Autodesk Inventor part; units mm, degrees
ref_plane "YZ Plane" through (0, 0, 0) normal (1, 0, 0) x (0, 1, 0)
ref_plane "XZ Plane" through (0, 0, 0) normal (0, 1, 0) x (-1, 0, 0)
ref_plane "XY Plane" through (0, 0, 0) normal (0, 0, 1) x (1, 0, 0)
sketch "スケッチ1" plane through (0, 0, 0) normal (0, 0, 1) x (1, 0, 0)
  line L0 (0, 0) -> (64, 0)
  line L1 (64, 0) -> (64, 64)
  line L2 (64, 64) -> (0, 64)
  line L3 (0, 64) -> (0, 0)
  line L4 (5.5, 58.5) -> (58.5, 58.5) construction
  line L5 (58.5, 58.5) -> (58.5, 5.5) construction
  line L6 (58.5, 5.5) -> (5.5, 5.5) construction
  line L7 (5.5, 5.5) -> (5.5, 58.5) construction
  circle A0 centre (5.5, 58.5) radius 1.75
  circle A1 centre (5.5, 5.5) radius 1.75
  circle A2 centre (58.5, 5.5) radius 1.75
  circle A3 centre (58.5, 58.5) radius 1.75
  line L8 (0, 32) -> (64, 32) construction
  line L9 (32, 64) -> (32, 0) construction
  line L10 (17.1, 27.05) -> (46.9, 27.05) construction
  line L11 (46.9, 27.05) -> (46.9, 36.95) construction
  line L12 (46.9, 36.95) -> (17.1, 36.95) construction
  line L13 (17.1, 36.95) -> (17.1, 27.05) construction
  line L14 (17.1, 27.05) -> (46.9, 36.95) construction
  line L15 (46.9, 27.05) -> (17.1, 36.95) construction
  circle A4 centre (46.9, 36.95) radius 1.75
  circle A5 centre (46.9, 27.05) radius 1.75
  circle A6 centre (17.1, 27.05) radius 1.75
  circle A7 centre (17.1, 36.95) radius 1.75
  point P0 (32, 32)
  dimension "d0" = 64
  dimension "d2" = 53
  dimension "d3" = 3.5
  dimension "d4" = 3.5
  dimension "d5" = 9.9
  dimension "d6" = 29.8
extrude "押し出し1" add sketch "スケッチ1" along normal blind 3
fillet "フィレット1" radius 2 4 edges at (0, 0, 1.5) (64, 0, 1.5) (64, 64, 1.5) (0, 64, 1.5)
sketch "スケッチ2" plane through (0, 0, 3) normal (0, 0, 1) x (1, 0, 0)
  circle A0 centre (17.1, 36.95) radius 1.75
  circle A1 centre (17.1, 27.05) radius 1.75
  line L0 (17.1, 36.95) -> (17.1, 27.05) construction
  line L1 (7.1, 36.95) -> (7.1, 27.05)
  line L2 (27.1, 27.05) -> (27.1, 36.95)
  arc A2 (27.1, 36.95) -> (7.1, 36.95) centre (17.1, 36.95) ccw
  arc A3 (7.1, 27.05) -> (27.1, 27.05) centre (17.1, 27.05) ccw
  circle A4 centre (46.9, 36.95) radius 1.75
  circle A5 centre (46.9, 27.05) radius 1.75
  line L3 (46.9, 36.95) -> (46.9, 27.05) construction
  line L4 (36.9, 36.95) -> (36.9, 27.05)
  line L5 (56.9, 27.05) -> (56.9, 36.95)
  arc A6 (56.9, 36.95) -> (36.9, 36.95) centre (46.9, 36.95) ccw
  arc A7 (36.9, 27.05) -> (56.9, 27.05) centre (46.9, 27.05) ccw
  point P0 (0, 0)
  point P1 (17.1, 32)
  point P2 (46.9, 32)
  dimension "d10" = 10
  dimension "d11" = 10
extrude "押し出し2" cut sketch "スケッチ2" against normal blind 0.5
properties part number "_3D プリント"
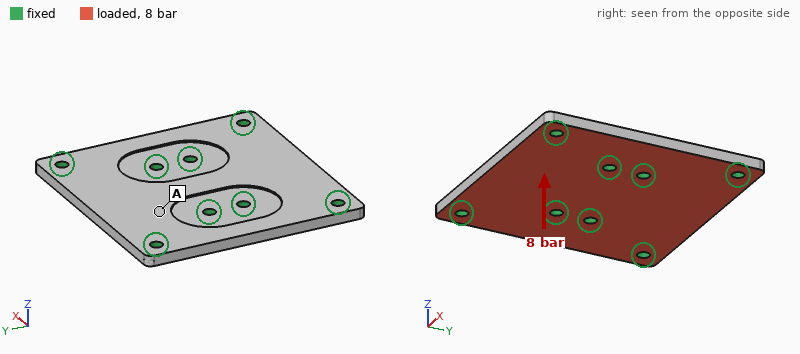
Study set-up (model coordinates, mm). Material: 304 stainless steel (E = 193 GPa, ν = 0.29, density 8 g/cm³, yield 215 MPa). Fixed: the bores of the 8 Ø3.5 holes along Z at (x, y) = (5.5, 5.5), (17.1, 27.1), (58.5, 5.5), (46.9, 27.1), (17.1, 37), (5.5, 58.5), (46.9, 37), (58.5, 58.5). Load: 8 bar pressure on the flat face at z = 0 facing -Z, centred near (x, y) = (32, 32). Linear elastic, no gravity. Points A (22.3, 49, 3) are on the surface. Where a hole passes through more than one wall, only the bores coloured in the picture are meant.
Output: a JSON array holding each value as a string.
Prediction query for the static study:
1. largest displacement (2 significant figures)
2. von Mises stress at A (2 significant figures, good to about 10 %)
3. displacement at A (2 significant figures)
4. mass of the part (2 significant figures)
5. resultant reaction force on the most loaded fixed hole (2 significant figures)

["31 µm", "16 MPa", "12 µm", "92 g", "420 N"]
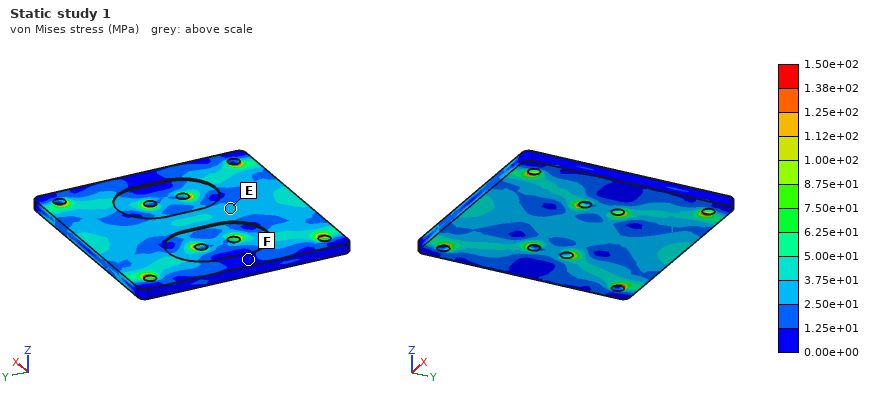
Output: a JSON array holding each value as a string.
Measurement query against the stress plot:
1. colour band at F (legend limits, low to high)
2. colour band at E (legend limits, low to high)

["0.00e+00 to 1.25e+01 MPa", "2.50e+01 to 3.75e+01 MPa"]
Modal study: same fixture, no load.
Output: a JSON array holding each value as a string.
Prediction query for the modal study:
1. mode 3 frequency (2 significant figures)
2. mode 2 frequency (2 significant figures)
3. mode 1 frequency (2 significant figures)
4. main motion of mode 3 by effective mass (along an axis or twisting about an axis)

["11 kHz", "6700 Hz", "6700 Hz", "twisting about Y"]
